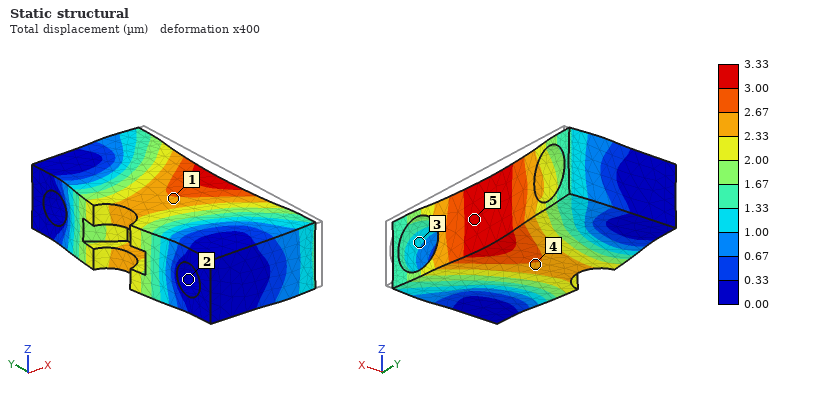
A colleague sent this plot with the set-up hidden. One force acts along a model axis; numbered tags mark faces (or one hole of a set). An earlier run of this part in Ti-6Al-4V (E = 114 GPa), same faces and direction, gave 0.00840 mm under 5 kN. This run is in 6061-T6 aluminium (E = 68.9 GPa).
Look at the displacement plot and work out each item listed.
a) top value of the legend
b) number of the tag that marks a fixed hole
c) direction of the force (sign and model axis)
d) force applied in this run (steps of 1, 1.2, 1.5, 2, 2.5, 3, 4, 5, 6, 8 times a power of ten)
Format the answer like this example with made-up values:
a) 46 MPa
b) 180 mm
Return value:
a) 3.33 µm
b) 2
c) -X
d) 1.2 kN
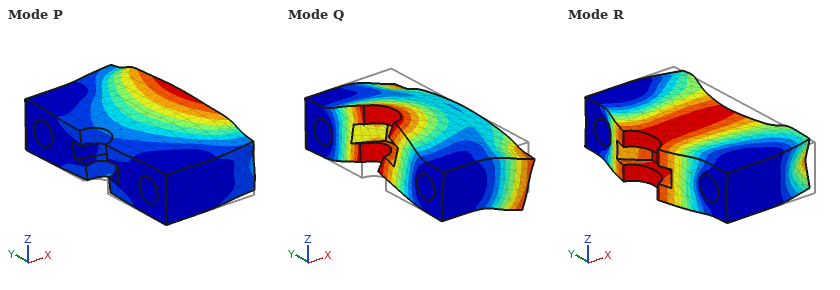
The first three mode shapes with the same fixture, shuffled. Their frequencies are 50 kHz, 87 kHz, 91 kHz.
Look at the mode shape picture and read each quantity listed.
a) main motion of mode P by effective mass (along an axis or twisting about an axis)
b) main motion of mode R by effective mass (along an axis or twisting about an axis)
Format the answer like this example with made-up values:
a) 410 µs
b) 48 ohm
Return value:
a) along Z
b) along X
